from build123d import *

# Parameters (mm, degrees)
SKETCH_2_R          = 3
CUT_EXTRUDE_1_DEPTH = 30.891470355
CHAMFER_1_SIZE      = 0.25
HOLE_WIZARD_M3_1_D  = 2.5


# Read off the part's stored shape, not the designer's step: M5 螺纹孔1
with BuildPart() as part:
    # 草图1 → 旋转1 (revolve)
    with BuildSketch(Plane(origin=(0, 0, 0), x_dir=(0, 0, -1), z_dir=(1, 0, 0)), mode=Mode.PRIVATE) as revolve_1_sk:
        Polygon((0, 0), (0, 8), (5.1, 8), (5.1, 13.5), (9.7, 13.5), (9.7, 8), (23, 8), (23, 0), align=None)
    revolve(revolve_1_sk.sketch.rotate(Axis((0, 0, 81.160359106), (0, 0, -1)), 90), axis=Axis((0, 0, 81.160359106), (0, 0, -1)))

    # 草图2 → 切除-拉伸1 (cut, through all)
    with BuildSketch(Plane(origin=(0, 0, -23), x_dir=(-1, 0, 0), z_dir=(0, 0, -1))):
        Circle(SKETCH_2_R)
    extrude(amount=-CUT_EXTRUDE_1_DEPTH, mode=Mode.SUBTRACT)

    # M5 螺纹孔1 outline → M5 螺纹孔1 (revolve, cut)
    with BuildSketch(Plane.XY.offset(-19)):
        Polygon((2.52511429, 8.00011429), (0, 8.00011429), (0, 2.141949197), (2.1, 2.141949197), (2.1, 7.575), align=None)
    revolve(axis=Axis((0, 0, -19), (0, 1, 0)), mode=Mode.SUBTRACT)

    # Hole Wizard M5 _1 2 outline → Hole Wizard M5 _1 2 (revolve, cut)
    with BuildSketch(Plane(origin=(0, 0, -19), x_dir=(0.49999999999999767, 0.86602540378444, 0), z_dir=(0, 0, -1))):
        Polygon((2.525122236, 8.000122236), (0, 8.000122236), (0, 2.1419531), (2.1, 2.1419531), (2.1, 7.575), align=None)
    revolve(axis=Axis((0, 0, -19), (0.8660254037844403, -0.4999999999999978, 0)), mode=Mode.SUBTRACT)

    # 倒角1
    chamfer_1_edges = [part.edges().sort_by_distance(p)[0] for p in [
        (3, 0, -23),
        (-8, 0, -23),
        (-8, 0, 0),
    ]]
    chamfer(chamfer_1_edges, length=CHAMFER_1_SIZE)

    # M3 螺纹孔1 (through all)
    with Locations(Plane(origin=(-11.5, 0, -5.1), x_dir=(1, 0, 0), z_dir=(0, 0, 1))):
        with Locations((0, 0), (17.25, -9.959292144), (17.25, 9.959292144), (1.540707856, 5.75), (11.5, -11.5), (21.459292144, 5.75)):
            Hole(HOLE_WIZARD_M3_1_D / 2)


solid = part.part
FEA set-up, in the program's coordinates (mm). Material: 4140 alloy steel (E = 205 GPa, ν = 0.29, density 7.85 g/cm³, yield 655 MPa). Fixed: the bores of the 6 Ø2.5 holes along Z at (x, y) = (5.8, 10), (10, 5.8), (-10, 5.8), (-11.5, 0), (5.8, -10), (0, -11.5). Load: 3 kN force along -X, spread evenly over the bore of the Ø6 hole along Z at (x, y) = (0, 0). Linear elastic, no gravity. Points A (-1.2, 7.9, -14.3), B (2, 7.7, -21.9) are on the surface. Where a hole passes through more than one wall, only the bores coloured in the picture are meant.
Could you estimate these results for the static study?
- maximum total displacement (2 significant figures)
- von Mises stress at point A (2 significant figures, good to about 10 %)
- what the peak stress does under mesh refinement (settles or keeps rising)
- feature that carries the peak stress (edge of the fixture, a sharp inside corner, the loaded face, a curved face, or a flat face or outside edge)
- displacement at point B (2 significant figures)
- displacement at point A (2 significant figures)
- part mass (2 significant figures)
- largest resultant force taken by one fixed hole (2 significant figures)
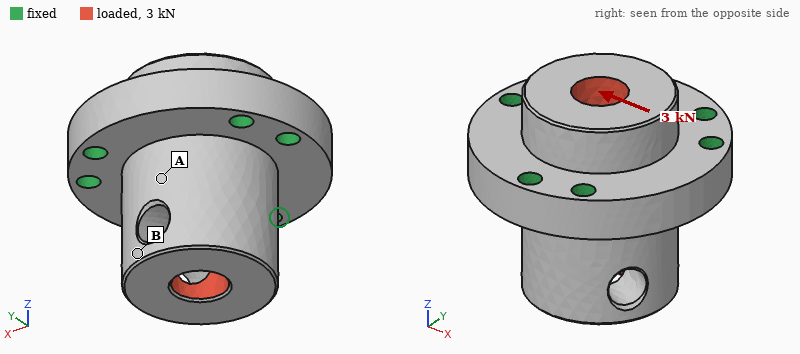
4.3 µm
15 MPa
keeps rising
edge of the fixture
3.6 µm
1.7 µm
42 g
760 N
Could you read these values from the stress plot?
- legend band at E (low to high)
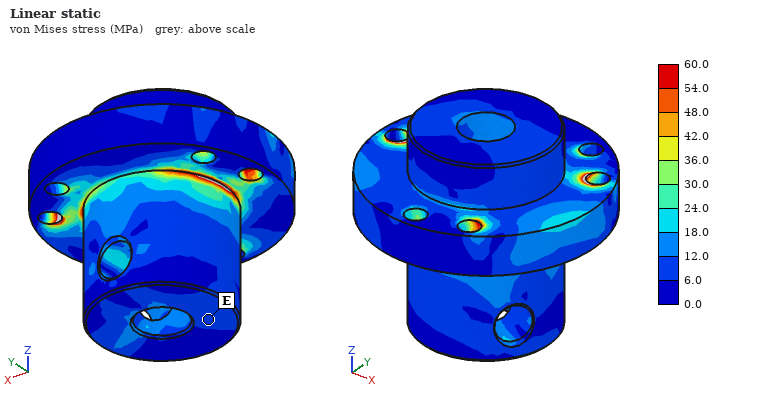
6.0 to 12.0 MPa
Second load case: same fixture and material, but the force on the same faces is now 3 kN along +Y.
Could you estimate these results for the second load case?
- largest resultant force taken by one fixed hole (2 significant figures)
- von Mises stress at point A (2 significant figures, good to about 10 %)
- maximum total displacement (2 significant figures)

760 N
10 MPa
4.2 µm
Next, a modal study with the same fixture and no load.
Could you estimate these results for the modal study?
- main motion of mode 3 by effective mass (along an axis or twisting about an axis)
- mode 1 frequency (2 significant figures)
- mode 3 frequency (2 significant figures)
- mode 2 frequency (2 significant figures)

along Z
27 kHz
40 kHz
27 kHz
